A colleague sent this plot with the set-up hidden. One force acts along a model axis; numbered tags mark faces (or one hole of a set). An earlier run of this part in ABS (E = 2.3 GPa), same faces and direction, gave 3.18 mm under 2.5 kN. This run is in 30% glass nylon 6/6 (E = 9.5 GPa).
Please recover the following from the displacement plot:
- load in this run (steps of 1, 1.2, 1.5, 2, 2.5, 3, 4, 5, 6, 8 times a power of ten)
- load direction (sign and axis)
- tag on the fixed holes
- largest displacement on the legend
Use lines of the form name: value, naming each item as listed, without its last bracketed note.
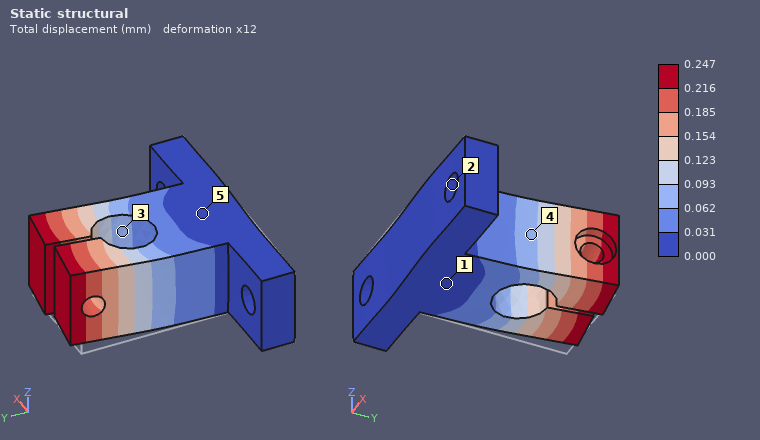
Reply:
load in this run: 800 N
load direction: +X
tag on the fixed holes: 2
largest displacement on the legend: 0.247 mm
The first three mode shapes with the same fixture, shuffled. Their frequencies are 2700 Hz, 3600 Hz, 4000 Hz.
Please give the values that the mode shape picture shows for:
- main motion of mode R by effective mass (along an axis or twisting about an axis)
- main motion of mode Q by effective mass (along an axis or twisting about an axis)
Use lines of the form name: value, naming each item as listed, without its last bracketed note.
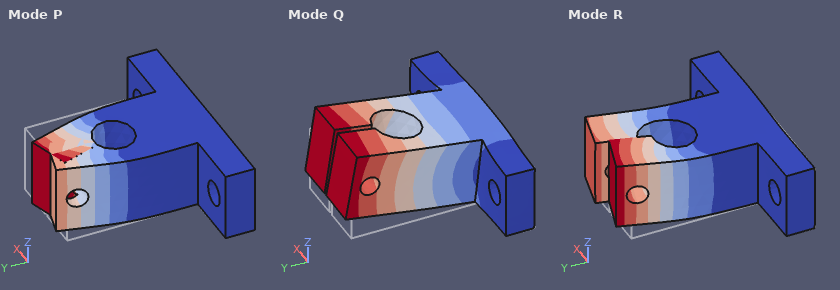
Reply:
main motion of mode R by effective mass: along X
main motion of mode Q by effective mass: along Z
